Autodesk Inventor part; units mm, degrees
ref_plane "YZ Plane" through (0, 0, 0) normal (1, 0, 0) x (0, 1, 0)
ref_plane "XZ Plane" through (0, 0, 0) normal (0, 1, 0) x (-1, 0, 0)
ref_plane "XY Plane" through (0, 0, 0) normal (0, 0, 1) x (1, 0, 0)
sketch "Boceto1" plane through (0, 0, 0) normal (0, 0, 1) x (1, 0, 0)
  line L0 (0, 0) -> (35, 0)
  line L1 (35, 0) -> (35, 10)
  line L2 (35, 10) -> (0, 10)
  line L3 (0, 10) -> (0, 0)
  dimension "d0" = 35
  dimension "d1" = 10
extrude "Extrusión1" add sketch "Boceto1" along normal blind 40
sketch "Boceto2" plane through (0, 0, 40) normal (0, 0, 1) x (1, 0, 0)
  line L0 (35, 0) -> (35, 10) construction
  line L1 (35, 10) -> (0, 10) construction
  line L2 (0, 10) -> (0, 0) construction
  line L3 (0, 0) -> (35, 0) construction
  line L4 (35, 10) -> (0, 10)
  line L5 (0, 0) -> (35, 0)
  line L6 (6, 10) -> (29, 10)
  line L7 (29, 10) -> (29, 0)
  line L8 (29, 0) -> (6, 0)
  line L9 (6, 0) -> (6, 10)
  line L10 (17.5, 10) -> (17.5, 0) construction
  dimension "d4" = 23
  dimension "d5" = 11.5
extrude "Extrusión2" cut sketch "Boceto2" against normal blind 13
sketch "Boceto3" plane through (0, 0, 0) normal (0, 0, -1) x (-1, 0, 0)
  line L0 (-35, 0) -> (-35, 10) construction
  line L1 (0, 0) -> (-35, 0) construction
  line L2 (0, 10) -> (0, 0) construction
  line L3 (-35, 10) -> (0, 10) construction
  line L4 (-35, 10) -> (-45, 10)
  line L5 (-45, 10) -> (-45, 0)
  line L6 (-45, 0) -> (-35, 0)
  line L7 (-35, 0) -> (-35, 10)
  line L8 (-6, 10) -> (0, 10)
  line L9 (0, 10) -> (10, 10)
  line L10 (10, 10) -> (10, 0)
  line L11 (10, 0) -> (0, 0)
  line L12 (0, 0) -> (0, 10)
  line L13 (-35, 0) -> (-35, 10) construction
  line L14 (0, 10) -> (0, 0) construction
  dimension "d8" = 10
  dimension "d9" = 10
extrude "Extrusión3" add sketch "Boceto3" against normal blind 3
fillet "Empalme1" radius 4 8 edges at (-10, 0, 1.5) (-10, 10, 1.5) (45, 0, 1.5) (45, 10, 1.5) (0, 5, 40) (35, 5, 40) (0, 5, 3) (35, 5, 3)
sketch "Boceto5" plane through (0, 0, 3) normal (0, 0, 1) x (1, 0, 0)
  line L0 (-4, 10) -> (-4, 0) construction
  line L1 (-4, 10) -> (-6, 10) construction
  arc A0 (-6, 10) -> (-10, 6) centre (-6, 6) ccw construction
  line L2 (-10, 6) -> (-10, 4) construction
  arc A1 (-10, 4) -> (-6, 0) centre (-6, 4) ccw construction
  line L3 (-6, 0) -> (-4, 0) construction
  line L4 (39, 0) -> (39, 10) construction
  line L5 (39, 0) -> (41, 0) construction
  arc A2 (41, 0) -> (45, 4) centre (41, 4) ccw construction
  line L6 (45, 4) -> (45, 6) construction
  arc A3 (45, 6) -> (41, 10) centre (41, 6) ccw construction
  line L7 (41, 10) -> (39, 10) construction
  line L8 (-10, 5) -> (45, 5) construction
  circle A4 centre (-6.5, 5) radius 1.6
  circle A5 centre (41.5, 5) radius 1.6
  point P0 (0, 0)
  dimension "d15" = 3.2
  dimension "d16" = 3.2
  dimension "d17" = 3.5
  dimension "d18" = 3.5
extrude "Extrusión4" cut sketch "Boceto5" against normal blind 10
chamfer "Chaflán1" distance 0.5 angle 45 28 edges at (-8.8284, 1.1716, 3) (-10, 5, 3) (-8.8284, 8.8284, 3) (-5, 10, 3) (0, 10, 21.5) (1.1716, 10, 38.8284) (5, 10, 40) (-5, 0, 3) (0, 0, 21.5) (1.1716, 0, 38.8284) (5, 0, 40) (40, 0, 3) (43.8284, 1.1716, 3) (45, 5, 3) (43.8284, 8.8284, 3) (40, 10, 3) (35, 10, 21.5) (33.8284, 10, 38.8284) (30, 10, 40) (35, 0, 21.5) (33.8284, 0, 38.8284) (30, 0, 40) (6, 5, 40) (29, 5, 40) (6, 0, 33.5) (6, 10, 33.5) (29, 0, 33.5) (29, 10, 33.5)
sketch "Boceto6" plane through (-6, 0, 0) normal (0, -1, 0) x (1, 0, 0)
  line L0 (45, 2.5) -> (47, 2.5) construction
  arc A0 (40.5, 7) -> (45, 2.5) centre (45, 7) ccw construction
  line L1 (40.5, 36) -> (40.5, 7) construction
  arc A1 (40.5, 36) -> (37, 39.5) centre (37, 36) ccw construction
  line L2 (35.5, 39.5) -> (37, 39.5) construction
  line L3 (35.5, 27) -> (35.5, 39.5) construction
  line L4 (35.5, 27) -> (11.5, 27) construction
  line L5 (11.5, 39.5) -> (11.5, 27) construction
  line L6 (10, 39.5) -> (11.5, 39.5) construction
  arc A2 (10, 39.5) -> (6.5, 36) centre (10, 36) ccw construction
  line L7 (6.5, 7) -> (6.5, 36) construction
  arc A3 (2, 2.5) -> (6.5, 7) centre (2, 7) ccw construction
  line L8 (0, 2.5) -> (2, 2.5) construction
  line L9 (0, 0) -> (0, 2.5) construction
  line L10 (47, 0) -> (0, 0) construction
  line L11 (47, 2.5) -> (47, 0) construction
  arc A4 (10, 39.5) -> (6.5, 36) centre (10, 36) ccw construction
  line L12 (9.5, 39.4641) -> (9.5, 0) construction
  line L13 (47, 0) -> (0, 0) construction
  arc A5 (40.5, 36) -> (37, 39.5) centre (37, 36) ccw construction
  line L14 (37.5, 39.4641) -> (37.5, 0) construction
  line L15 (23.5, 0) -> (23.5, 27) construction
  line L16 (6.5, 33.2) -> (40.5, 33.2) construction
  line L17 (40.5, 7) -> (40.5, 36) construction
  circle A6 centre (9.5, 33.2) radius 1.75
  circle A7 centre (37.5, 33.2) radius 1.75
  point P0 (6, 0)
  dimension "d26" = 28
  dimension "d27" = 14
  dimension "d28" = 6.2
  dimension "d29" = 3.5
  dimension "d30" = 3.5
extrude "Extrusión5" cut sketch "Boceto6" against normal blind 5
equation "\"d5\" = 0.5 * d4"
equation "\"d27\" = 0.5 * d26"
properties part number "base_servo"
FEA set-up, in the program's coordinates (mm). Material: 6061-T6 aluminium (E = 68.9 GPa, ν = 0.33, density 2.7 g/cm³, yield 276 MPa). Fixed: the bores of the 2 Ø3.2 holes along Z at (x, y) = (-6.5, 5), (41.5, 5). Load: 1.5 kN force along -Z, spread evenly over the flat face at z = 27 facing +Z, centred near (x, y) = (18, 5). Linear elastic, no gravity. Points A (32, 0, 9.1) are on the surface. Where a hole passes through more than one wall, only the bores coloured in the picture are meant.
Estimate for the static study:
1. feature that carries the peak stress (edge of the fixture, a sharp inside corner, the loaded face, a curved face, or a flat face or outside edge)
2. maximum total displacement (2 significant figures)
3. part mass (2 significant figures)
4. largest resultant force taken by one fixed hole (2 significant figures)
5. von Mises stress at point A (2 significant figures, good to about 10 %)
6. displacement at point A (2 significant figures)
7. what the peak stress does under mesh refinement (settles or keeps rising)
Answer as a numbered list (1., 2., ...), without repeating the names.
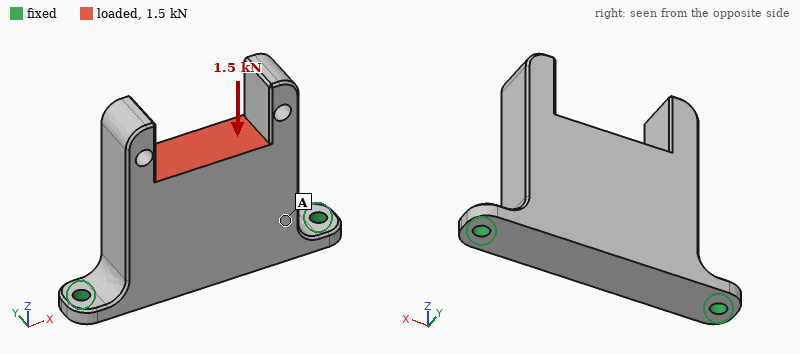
1. edge of the fixture
2. 19 µm
3. 31 g
4. 930 N
5. 17 MPa
6. 17 µm
7. keeps rising
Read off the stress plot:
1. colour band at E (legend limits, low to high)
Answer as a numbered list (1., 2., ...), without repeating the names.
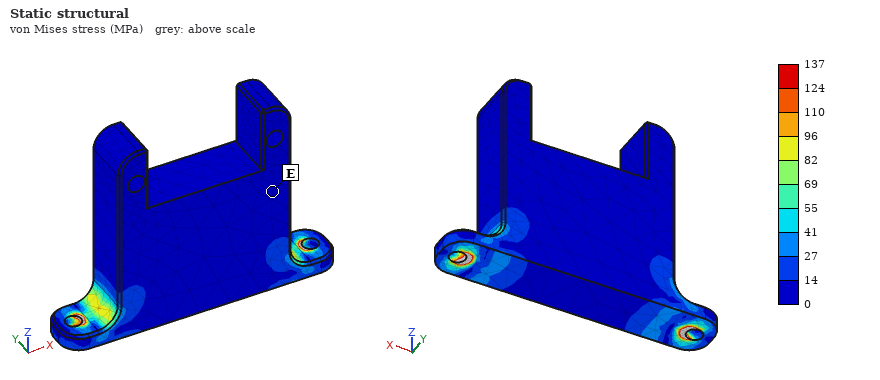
1. 0 to 14 MPa
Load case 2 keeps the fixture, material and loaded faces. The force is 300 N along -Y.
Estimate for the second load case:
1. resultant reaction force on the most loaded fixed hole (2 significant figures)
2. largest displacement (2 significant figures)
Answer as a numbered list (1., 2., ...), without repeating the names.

1. 150 N
2. 0.32 mm
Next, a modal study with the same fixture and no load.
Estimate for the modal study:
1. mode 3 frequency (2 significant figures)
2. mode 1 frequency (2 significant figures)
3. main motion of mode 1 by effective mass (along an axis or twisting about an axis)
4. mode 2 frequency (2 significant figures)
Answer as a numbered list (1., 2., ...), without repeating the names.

1. 8500 Hz
2. 1600 Hz
3. along Y
4. 8300 Hz
